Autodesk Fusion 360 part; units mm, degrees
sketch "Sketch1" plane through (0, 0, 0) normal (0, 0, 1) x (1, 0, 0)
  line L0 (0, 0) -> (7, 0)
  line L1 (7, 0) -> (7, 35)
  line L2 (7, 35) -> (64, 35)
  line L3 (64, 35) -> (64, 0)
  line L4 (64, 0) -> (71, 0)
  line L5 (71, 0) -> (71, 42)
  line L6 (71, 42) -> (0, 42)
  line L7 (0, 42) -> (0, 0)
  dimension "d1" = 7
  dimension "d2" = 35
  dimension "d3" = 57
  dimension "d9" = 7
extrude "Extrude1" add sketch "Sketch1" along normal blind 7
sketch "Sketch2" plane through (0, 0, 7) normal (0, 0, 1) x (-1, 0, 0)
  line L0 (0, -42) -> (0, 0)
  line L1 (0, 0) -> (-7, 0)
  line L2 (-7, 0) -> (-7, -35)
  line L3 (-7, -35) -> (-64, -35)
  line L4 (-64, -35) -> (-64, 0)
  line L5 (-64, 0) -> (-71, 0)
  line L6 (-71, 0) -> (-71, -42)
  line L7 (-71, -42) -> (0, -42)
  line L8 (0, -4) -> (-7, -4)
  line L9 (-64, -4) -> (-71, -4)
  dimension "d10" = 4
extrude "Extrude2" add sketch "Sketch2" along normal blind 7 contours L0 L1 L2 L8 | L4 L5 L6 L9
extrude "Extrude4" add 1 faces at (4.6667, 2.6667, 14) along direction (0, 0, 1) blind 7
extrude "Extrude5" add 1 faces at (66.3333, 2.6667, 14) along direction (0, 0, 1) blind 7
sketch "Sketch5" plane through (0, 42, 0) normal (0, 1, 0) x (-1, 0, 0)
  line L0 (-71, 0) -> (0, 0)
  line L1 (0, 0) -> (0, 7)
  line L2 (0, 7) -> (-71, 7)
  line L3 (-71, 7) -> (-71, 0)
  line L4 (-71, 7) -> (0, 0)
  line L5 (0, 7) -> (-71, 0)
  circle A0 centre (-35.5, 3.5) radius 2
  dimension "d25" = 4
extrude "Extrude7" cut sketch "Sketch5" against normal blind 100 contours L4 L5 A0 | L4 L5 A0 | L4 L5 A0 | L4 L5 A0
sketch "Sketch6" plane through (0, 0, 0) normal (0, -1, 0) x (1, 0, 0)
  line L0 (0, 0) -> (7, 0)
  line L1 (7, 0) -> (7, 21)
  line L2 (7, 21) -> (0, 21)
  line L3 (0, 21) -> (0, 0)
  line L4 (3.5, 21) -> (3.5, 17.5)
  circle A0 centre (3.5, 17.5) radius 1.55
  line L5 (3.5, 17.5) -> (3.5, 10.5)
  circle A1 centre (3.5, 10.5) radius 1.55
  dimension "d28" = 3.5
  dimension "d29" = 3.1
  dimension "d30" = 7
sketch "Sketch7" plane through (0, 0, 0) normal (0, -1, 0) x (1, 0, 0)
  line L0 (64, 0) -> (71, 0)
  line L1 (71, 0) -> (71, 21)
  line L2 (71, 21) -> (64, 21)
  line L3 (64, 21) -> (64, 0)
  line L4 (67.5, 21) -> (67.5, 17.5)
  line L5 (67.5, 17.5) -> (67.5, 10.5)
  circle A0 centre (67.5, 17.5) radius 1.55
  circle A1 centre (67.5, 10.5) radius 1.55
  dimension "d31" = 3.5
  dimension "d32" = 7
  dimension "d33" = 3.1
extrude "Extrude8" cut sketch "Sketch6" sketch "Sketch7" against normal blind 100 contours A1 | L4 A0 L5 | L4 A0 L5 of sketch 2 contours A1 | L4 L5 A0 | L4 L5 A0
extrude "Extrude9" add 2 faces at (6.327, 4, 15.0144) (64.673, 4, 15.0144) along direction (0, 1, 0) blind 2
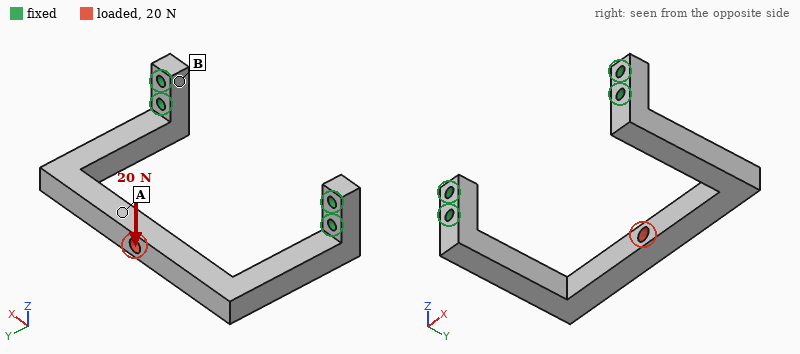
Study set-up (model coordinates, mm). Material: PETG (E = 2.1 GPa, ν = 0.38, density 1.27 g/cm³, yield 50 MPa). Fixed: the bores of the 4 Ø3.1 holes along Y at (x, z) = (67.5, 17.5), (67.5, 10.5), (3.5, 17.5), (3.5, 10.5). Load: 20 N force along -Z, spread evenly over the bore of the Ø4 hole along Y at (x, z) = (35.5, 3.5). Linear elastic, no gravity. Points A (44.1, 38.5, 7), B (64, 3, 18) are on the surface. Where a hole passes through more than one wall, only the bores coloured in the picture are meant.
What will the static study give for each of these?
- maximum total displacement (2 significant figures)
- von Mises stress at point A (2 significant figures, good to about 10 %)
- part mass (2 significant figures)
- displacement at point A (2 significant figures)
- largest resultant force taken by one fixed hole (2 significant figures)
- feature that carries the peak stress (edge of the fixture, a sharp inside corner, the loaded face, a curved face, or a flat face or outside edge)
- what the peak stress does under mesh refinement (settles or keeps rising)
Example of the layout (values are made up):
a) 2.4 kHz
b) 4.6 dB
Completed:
a) 0.86 mm
b) 3.1 MPa
c) 9.9 g
d) 0.75 mm
e) 10 N
f) edge of the fixture
g) keeps rising
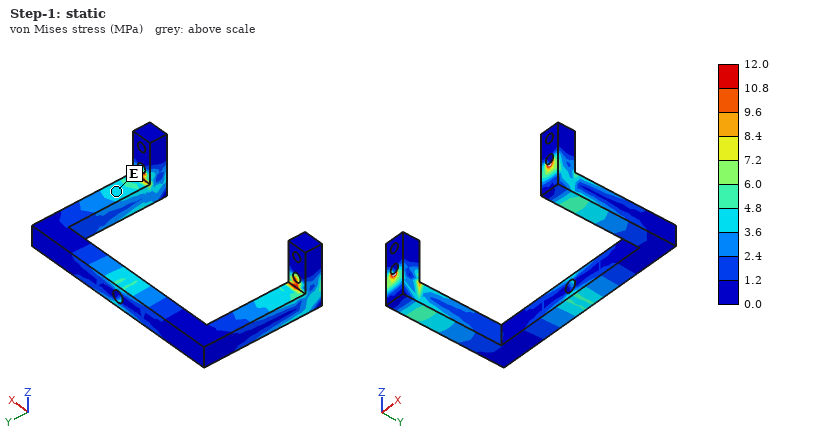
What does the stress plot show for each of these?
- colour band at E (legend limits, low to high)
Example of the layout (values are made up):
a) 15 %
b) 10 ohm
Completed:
a) 3.6 to 4.8 MPa
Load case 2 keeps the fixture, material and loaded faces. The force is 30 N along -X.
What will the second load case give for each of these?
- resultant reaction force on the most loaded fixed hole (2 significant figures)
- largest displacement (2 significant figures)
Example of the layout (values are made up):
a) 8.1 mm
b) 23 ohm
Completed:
a) 20 N
b) 0.35 mm
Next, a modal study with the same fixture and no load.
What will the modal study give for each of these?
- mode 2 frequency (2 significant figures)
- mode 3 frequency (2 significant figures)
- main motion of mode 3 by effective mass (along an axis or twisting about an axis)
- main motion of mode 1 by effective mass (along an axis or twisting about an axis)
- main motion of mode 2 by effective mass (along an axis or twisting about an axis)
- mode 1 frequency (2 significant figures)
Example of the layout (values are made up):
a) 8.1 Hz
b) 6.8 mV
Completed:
a) 640 Hz
b) 760 Hz
c) twisting about Y
d) along Z
e) along X
f) 400 Hz
